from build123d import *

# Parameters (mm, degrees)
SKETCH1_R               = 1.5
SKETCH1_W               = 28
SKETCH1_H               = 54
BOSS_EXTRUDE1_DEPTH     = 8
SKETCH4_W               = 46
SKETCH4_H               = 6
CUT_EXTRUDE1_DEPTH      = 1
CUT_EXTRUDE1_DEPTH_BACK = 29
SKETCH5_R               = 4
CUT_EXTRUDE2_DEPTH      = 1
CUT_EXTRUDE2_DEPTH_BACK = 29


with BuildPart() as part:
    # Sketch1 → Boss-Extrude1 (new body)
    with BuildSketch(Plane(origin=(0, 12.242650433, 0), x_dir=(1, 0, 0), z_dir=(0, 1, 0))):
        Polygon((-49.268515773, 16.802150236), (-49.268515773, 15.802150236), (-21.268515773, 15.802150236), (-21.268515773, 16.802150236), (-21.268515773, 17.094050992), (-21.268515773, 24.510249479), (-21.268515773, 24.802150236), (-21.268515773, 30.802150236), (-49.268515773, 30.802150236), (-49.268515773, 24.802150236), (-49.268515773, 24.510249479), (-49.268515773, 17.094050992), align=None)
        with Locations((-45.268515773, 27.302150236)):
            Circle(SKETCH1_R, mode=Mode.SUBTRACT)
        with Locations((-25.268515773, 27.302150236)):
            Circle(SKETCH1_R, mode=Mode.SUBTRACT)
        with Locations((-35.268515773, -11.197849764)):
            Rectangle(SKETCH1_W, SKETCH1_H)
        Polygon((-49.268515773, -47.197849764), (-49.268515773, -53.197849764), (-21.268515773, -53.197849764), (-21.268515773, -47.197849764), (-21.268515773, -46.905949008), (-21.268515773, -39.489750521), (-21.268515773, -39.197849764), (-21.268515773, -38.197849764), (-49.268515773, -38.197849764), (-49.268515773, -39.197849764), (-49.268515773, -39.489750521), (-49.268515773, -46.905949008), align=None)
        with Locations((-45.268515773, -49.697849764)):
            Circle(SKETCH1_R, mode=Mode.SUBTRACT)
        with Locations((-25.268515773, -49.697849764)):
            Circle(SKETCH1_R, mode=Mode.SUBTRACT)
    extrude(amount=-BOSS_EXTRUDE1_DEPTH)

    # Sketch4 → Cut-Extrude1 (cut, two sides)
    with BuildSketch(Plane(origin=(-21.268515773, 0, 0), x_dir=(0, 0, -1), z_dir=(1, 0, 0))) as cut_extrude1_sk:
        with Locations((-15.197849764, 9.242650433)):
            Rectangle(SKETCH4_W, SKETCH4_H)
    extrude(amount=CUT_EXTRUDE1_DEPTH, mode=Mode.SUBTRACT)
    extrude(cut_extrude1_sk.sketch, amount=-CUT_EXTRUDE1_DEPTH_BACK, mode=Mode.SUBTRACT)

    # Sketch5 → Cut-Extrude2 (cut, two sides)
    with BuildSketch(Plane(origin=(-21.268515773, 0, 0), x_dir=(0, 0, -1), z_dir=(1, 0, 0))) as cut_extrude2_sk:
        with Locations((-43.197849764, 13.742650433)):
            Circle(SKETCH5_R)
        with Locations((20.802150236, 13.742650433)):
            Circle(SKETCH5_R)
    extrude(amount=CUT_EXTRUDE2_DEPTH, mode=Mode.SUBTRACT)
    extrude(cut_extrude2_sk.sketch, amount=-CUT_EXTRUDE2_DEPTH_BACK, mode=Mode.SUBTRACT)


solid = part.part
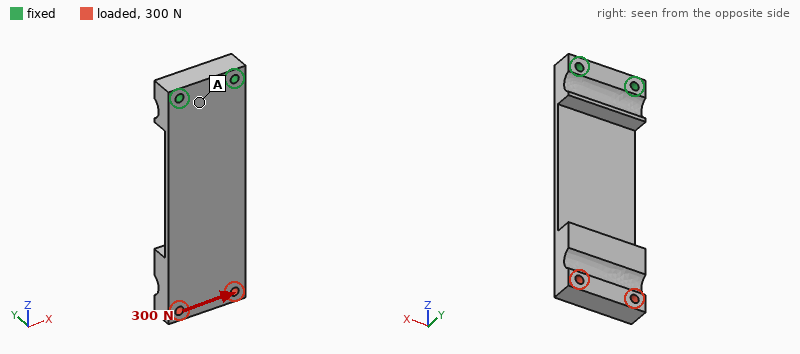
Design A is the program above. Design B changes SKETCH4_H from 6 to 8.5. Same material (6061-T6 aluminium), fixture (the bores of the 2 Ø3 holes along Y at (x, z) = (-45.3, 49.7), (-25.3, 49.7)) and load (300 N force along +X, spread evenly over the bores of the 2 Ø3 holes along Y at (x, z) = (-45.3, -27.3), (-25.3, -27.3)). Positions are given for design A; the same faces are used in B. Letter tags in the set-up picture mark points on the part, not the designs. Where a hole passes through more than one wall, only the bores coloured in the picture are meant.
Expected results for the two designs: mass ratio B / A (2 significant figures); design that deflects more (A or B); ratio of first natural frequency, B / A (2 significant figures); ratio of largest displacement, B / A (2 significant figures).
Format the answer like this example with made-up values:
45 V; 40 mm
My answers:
0.84; B; 0.25; 14
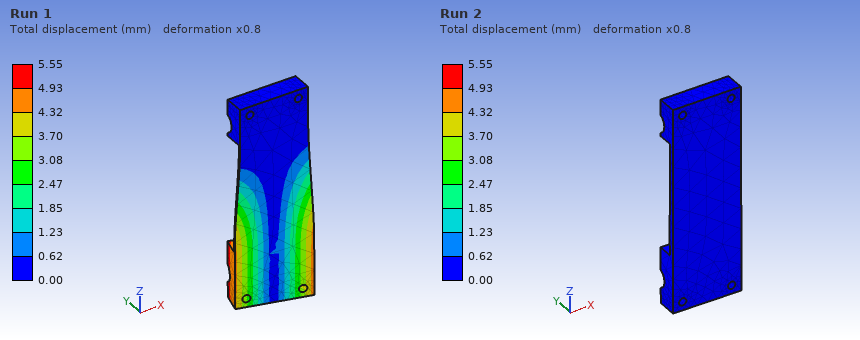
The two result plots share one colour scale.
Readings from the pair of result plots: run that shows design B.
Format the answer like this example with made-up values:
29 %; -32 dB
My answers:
Run 1
